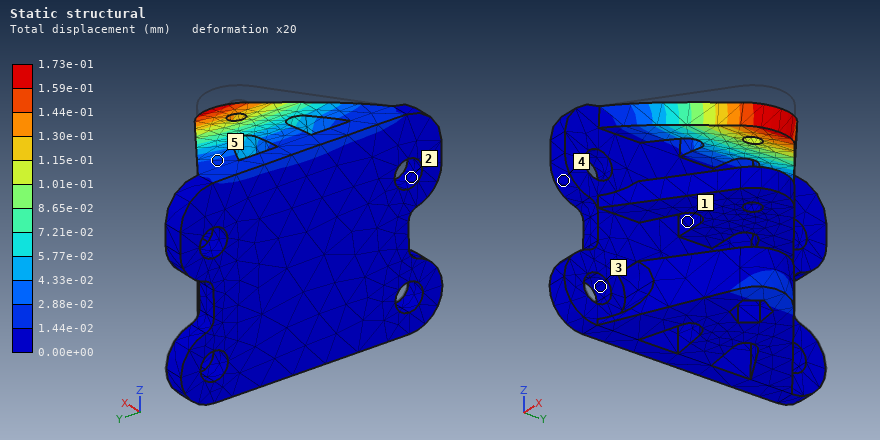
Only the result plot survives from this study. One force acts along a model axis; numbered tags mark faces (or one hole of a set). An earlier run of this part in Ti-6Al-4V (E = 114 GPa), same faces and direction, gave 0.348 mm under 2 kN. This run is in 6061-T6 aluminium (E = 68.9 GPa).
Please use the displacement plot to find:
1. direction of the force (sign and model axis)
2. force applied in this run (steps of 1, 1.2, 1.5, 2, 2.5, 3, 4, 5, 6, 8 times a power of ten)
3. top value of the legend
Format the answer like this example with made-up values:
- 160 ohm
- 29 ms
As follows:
- -Z
- 600 N
- 1.73e-01 mm
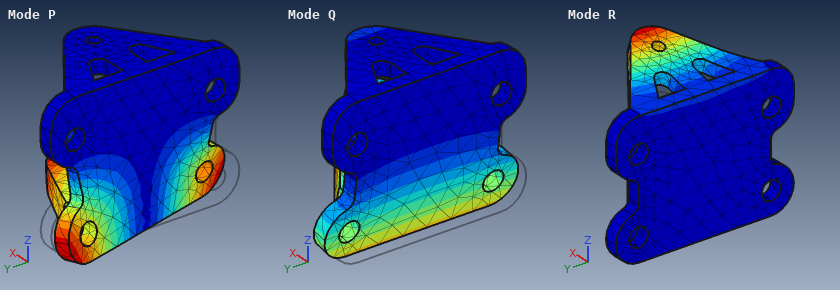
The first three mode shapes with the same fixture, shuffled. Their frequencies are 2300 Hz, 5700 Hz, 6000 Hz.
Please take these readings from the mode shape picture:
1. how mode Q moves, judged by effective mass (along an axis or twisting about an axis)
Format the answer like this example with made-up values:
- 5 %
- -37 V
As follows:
- along X
